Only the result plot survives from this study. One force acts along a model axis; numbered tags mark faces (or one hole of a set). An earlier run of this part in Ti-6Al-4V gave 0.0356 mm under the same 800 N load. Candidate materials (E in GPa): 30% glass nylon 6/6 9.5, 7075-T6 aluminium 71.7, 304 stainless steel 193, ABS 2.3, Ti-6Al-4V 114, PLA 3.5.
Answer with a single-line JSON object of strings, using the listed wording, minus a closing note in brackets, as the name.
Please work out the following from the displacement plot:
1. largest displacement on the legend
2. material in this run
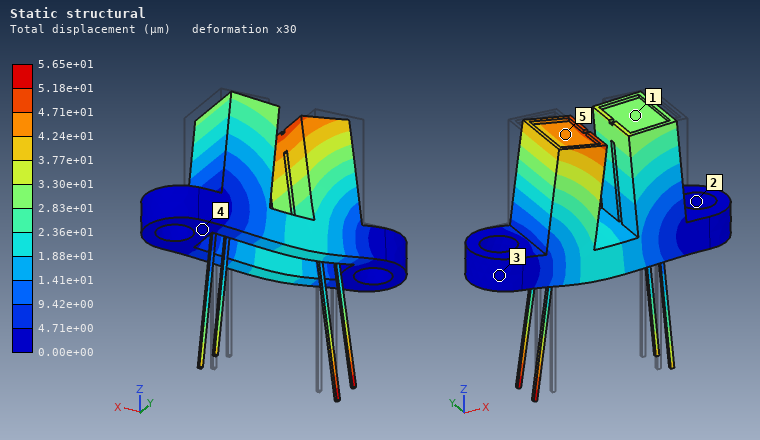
{"largest displacement on the legend": "5.65e+01 µm", "material in this run": "7075-T6 aluminium"}
